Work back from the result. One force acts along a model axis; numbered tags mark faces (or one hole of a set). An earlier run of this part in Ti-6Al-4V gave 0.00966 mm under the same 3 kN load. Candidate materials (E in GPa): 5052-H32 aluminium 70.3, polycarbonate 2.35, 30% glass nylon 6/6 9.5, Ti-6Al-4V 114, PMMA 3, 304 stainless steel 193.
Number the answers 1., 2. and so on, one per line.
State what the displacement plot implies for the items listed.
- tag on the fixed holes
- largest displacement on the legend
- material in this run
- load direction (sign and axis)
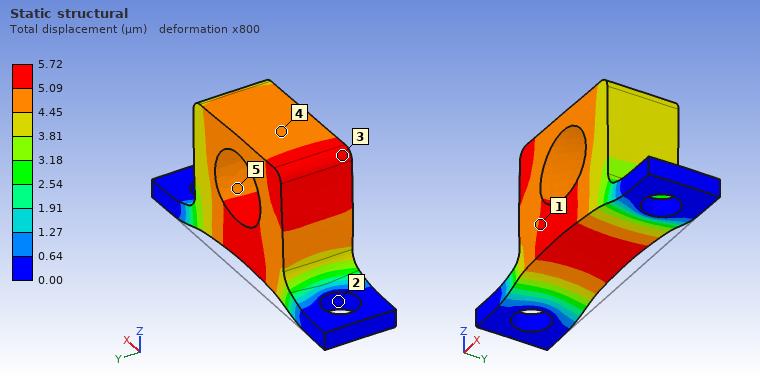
1. 2
2. 5.72 µm
3. 304 stainless steel
4. +Z
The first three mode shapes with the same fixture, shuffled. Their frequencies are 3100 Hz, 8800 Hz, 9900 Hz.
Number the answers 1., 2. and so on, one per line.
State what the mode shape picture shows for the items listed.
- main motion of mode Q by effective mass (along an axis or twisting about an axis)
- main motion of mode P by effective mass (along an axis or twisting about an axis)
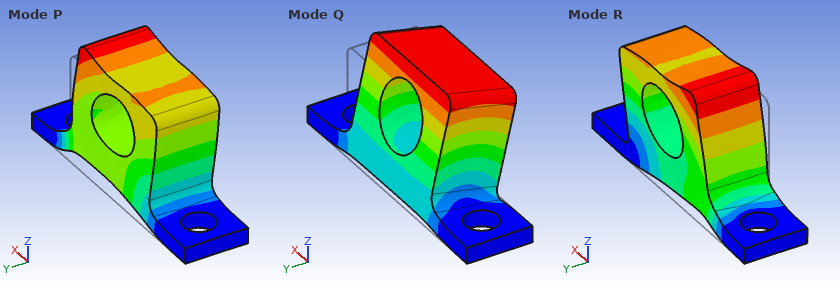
1. along Y
2. along Z
